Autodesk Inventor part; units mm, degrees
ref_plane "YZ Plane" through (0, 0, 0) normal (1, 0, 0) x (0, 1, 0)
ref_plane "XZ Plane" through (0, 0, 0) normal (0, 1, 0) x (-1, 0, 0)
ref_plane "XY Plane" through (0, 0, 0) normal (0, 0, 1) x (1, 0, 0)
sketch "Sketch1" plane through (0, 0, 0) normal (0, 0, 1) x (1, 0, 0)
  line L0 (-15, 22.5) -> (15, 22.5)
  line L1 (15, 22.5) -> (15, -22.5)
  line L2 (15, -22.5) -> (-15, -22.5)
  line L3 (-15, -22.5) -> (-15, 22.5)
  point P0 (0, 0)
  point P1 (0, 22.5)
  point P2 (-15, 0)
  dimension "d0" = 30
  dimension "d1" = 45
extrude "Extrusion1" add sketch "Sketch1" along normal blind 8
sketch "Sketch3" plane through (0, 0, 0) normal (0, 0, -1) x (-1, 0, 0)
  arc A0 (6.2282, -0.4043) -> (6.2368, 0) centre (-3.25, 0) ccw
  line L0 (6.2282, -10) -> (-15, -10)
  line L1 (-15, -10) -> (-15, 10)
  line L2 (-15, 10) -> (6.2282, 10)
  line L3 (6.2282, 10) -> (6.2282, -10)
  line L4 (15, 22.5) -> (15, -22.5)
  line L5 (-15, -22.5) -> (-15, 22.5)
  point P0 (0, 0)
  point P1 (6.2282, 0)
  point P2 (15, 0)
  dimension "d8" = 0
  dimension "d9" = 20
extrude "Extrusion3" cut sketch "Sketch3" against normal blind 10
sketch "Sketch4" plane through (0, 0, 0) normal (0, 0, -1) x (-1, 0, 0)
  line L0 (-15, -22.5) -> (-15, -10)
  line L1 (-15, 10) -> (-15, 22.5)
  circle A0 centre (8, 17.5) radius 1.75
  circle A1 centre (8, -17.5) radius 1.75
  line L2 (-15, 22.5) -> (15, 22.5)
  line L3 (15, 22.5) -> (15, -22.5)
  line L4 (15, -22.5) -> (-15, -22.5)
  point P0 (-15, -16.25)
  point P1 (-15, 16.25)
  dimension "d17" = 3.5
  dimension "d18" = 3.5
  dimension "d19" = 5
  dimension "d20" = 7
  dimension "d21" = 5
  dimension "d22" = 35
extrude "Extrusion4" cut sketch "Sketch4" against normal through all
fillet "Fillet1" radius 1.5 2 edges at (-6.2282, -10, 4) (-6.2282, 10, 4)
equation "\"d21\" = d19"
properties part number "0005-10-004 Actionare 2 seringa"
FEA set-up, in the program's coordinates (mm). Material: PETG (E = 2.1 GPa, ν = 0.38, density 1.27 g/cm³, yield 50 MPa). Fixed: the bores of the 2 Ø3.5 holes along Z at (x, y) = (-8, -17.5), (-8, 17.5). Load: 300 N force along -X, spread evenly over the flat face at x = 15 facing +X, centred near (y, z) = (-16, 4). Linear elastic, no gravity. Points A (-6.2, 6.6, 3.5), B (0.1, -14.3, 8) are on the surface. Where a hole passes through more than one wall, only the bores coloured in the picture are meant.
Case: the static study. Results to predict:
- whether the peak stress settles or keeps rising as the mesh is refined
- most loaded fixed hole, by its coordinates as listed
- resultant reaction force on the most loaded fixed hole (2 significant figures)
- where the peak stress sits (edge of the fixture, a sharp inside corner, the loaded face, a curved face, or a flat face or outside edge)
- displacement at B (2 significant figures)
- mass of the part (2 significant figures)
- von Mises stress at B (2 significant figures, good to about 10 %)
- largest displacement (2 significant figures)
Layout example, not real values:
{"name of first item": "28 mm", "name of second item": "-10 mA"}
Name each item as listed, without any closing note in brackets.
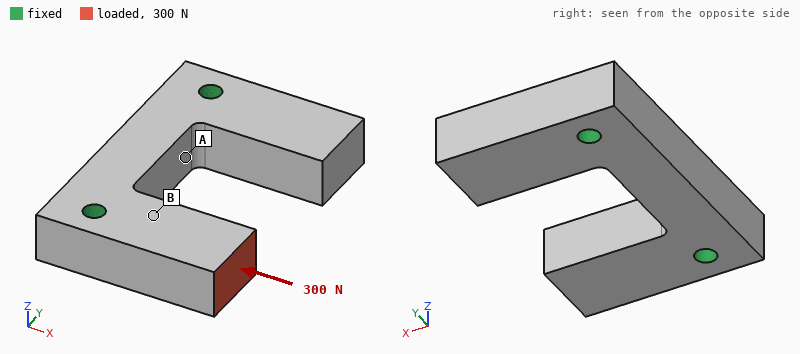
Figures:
{"whether the peak stress settles or keeps rising as the mesh is refined": "keeps rising", "most loaded fixed hole, by its coordinates as listed": "(-8, -17.5)", "resultant reaction force on the most loaded fixed hole": "290 N", "where the peak stress sits": "edge of the fixture", "displacement at B": "18 µm", "mass of the part": "9.2 g", "von Mises stress at B": "3.2 MPa", "largest displacement": "48 µm"}
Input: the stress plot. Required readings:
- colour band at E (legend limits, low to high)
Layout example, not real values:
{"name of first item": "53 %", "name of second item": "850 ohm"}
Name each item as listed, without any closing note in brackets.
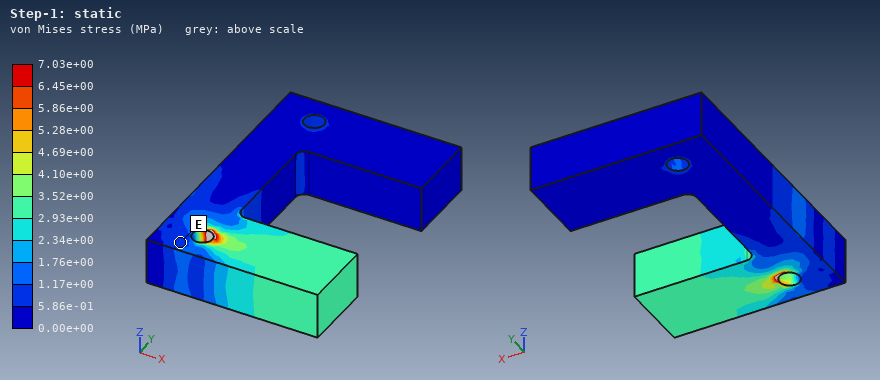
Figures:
{"colour band at E": "5.86e-01 to 1.17e+00 MPa"}
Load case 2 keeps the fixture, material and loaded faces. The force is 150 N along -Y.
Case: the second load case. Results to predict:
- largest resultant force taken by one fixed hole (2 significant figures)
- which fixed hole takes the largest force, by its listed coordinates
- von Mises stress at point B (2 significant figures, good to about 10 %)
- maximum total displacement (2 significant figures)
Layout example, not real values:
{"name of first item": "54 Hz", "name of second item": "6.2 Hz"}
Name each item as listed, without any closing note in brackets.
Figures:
{"largest resultant force taken by one fixed hole": "210 N", "which fixed hole takes the largest force, by its listed coordinates": "(-8, -17.5)", "von Mises stress at point B": "4.9 MPa", "maximum total displacement": "0.45 mm"}
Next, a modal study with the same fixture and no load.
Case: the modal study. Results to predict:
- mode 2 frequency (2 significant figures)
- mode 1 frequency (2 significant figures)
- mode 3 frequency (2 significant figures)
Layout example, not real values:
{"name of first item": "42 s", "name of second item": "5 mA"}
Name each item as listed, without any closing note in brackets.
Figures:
{"mode 2 frequency": "2900 Hz", "mode 1 frequency": "2900 Hz", "mode 3 frequency": "2900 Hz"}
